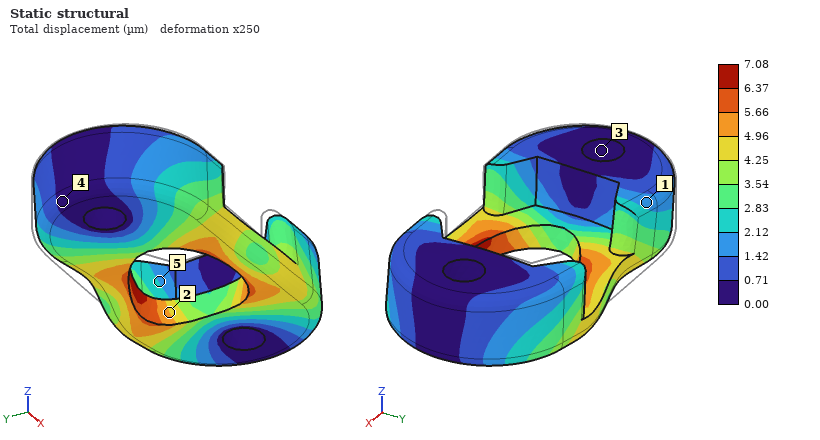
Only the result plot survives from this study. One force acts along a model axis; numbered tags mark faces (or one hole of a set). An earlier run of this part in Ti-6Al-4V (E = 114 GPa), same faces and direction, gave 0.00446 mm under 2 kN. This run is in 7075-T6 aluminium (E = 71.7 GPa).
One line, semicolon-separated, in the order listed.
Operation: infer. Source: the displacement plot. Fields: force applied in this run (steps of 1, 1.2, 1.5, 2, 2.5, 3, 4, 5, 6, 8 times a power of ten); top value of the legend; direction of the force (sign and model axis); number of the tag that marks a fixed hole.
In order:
2 kN; 7.08 µm; +X; 3
